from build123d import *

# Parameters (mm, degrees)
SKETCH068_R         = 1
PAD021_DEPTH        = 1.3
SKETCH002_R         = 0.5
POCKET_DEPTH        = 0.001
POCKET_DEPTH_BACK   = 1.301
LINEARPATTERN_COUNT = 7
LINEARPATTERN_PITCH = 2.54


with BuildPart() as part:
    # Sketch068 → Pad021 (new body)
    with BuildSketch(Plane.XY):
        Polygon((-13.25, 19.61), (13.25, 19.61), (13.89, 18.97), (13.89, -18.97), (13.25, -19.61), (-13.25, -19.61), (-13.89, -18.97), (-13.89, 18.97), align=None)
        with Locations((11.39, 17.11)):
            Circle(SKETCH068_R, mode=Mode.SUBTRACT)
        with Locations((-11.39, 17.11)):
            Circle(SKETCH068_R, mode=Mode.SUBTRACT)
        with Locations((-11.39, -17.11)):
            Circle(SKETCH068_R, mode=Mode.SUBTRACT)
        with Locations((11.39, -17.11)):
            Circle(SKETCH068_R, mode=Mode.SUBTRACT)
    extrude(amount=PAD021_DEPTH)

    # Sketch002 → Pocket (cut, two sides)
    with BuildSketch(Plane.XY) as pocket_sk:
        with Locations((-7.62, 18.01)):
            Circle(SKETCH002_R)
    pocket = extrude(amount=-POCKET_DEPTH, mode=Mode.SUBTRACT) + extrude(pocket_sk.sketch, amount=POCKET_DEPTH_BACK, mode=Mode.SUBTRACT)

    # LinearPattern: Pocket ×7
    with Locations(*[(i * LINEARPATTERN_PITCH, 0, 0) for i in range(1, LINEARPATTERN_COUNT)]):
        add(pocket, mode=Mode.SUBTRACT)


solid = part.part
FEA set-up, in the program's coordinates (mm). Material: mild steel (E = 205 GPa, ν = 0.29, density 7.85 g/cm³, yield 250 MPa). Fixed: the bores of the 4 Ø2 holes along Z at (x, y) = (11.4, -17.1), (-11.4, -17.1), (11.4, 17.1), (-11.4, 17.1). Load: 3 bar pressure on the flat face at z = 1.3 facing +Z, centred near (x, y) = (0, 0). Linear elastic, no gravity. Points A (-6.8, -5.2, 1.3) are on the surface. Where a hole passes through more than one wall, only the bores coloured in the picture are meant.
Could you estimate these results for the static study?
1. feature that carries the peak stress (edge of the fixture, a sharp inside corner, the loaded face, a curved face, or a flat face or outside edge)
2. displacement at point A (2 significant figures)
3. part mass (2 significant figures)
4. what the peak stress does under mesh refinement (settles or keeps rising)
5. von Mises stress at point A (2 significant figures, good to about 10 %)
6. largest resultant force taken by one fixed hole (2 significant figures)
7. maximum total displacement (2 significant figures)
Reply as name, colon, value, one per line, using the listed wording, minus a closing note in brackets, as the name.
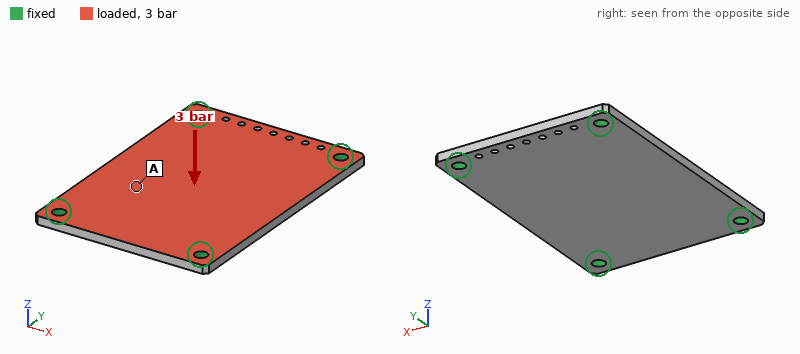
feature that carries the peak stress: edge of the fixture
displacement at point A: 33 µm
part mass: 11 g
what the peak stress does under mesh refinement: keeps rising
von Mises stress at point A: 43 MPa
largest resultant force taken by one fixed hole: 81 N
maximum total displacement: 41 µm
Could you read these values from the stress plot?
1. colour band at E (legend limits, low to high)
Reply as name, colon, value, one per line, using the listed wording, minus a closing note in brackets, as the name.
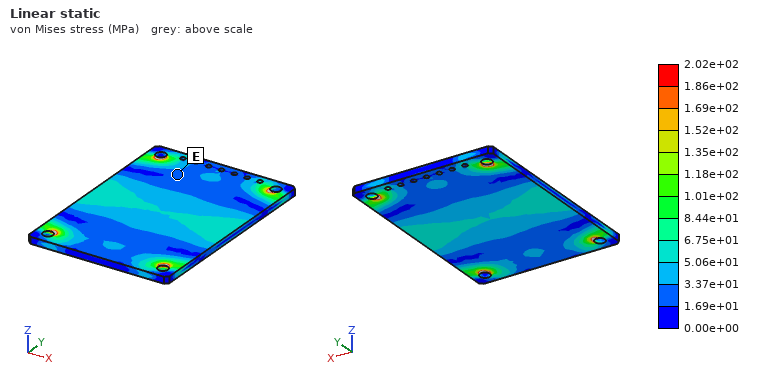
colour band at E: 1.69e+01 to 3.37e+01 MPa
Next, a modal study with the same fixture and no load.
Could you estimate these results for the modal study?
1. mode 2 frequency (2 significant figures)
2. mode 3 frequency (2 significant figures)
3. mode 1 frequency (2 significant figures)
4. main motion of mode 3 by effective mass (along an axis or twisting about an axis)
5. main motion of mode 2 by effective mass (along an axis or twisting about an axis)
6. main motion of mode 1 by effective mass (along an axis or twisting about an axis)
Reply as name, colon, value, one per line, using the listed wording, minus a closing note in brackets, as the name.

mode 2 frequency: 7700 Hz
mode 3 frequency: 12 kHz
mode 1 frequency: 5000 Hz
main motion of mode 3 by effective mass: twisting about X
main motion of mode 2 by effective mass: twisting about Y
main motion of mode 1 by effective mass: along Z
